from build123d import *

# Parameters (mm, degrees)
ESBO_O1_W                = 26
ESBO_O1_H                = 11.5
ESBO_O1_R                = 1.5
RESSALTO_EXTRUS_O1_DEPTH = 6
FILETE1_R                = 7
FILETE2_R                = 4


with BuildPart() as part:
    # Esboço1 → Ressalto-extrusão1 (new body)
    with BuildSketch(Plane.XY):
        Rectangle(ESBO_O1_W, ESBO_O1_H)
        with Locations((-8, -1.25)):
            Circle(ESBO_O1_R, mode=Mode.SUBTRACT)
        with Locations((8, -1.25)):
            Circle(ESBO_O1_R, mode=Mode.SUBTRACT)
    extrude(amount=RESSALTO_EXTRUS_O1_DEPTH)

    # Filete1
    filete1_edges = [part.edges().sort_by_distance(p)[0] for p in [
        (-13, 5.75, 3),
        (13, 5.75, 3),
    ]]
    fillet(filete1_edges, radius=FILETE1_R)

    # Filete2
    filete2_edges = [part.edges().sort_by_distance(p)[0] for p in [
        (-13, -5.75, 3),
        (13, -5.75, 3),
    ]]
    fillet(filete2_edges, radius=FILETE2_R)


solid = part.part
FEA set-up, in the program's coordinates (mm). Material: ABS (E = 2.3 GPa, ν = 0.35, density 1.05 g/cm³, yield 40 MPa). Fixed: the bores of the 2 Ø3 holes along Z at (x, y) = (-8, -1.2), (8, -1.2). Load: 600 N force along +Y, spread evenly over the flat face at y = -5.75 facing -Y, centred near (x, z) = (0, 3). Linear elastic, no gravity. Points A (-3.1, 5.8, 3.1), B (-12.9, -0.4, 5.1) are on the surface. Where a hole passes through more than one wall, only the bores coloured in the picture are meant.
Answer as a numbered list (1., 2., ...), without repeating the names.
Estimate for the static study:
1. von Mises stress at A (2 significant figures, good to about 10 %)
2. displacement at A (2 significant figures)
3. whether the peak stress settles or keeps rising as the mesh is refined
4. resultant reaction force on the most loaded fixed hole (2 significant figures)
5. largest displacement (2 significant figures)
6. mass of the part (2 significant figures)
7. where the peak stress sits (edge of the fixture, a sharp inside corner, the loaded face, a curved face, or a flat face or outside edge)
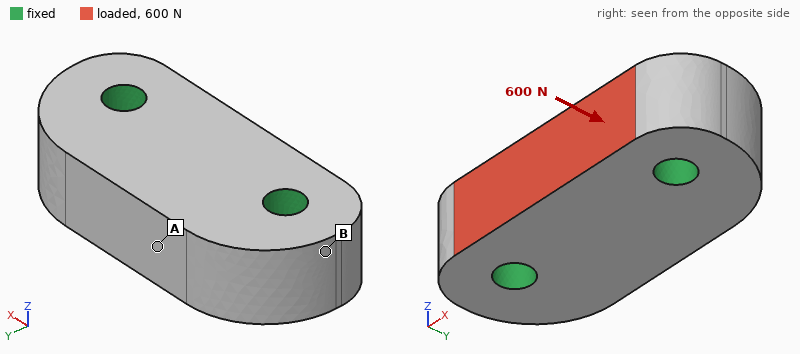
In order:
1. 4.0 MPa
2. 17 µm
3. keeps rising
4. 300 N
5. 34 µm
6. 1.6 g
7. edge of the fixture
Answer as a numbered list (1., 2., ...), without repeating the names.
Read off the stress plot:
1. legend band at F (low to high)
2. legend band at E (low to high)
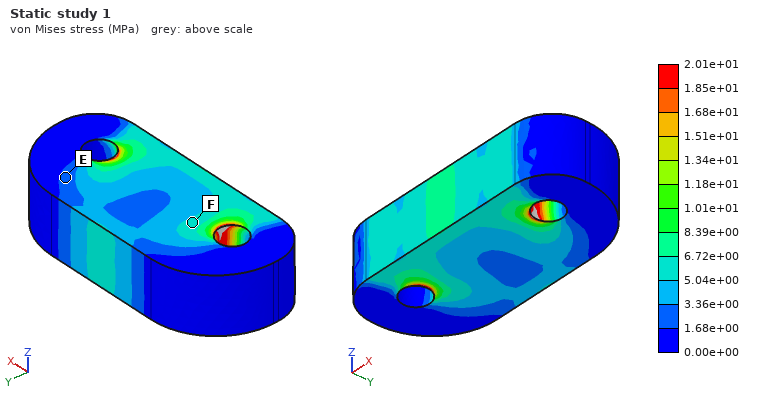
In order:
1. 5.04e+00 to 6.72e+00 MPa
2. 1.68e+00 to 3.36e+00 MPa
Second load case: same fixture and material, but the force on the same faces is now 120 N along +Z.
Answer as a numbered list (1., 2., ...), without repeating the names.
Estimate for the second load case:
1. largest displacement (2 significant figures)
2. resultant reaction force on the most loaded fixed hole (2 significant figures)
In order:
1. 26 µm
2. 60 N
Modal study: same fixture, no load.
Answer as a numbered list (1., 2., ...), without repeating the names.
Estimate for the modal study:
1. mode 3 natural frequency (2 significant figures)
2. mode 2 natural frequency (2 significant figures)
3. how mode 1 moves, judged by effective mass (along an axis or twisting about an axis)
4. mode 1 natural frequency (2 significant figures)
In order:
1. 23 kHz
2. 23 kHz
3. along Z
4. 17 kHz
